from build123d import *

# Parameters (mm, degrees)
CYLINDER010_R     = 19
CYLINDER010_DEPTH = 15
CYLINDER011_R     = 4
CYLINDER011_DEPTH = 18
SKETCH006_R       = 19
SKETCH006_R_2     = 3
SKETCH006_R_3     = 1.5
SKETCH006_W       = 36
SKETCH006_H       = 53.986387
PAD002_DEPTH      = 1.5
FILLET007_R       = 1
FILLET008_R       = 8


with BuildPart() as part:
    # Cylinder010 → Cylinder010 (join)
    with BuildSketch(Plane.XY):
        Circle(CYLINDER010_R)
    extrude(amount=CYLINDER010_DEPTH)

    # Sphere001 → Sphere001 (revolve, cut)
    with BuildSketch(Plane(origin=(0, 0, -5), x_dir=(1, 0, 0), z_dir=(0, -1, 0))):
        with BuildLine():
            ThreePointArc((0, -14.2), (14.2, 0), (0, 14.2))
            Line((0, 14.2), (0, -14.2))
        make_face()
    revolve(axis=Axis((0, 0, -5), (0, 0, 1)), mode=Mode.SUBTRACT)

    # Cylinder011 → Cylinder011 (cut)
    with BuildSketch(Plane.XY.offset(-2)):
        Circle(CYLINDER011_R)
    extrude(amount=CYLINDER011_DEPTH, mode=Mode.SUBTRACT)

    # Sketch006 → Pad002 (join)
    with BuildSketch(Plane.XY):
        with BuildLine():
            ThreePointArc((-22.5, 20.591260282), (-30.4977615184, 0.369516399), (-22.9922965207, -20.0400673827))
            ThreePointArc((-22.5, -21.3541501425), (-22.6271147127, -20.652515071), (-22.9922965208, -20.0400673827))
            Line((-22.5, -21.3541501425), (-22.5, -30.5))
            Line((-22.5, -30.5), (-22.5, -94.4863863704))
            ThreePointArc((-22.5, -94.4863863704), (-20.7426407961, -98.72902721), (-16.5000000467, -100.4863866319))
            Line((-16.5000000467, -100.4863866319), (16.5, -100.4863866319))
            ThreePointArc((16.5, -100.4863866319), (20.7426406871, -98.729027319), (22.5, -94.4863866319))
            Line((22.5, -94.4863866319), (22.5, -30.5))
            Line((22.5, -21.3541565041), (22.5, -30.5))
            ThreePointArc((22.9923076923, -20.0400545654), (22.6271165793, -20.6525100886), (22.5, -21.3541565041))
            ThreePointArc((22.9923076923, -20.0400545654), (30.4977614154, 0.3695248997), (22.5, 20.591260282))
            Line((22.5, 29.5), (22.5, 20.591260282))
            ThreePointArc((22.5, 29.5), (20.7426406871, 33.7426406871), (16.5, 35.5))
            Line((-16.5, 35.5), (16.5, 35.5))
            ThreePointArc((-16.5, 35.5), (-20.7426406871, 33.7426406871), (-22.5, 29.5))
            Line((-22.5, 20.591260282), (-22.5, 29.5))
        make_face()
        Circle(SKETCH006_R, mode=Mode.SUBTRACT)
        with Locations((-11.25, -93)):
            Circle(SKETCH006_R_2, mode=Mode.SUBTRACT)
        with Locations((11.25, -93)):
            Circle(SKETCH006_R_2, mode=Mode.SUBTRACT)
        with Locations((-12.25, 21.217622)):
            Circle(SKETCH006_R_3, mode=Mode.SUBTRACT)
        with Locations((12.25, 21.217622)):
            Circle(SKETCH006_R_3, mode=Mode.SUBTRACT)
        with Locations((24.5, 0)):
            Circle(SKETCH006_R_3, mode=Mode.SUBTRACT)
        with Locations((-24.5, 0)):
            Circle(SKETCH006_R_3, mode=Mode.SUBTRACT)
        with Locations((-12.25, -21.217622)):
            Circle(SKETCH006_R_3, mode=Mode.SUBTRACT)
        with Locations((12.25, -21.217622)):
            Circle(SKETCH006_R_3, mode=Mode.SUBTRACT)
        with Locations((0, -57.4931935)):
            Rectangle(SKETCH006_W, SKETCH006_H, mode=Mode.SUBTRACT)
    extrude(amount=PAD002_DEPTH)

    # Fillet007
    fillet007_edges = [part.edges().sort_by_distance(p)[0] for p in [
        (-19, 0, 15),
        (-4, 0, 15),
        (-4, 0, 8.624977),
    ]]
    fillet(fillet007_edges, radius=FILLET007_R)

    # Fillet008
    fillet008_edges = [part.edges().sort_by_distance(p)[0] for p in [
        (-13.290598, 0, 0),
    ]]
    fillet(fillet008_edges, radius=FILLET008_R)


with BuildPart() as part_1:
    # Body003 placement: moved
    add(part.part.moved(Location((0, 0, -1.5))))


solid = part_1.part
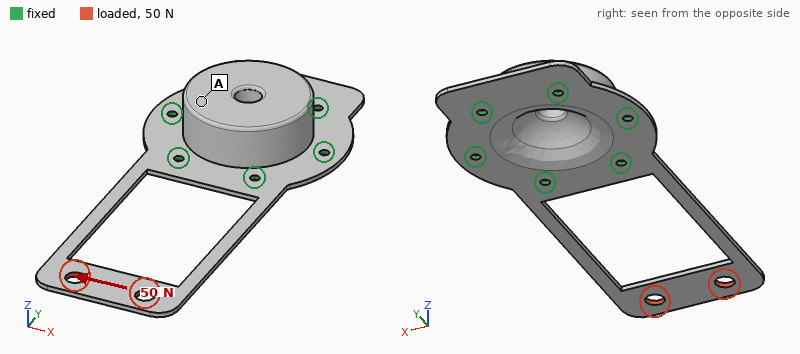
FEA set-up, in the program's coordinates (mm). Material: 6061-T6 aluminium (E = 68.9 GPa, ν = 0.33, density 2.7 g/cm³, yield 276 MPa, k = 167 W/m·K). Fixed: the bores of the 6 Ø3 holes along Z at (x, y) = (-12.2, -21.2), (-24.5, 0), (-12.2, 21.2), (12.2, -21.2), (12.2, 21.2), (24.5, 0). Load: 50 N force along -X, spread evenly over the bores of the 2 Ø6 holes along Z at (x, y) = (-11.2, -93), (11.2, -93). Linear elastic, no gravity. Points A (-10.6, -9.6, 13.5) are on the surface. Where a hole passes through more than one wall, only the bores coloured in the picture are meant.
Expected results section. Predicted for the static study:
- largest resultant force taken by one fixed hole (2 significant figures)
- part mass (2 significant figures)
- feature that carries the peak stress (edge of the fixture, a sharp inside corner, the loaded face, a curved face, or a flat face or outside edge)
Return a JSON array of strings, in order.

["42 N", "50 g", "a flat face or outside edge"]
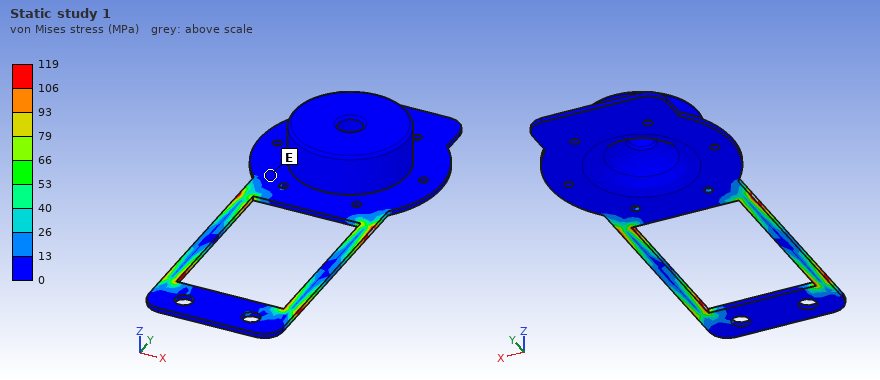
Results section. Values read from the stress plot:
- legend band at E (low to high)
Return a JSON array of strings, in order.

["0 to 13 MPa"]
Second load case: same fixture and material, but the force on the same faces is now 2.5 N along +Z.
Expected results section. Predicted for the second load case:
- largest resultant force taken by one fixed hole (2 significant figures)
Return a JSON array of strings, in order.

["2.7 N"]
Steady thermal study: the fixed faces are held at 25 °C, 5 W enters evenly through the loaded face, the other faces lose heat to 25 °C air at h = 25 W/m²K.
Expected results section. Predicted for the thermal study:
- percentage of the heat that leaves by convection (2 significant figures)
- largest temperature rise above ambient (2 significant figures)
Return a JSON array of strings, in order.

["65 %", "65 K"]
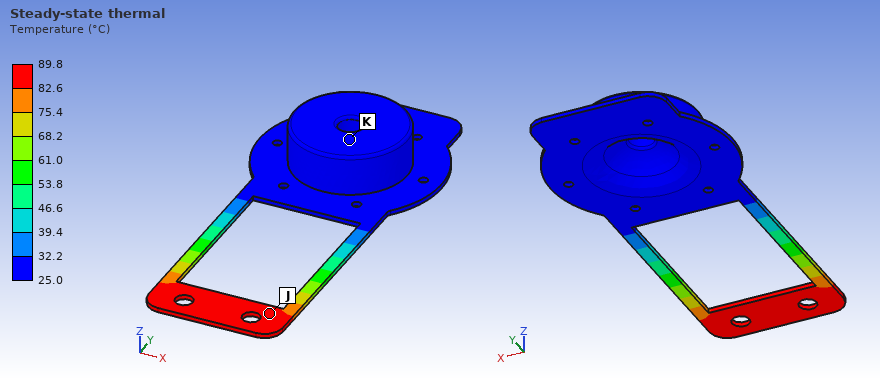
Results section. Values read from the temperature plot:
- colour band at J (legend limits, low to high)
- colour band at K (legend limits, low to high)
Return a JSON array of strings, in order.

["82.6 to 89.8 °C", "25.0 to 32.2 °C"]
